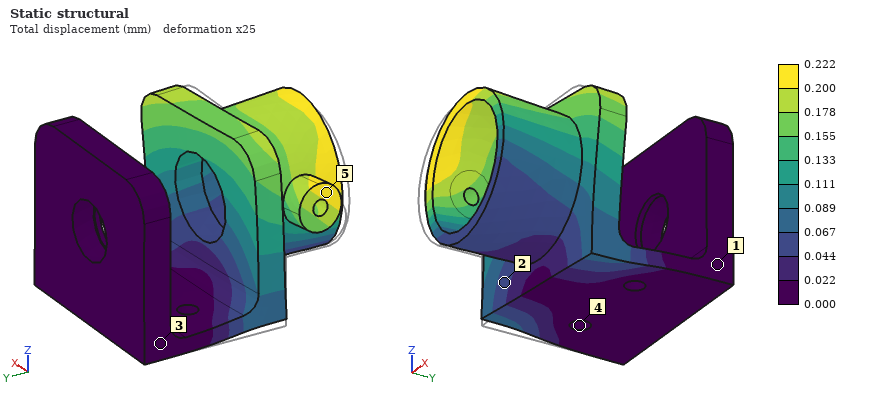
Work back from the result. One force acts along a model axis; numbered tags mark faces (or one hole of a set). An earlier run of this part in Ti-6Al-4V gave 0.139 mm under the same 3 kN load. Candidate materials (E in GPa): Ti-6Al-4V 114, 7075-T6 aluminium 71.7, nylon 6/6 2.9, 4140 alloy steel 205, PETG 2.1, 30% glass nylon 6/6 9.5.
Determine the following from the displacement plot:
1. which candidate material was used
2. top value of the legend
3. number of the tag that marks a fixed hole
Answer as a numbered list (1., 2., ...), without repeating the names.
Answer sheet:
1. 7075-T6 aluminium
2. 0.222 mm
3. 4
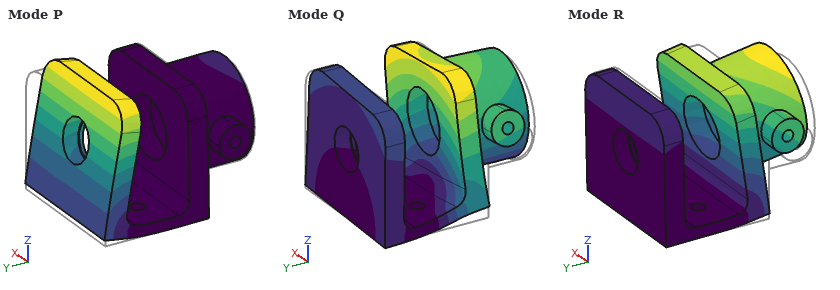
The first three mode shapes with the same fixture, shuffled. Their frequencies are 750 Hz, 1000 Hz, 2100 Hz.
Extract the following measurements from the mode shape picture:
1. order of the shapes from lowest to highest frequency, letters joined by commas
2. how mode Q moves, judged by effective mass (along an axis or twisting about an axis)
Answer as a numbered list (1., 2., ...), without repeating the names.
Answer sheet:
1. R, P, Q
2. along X
